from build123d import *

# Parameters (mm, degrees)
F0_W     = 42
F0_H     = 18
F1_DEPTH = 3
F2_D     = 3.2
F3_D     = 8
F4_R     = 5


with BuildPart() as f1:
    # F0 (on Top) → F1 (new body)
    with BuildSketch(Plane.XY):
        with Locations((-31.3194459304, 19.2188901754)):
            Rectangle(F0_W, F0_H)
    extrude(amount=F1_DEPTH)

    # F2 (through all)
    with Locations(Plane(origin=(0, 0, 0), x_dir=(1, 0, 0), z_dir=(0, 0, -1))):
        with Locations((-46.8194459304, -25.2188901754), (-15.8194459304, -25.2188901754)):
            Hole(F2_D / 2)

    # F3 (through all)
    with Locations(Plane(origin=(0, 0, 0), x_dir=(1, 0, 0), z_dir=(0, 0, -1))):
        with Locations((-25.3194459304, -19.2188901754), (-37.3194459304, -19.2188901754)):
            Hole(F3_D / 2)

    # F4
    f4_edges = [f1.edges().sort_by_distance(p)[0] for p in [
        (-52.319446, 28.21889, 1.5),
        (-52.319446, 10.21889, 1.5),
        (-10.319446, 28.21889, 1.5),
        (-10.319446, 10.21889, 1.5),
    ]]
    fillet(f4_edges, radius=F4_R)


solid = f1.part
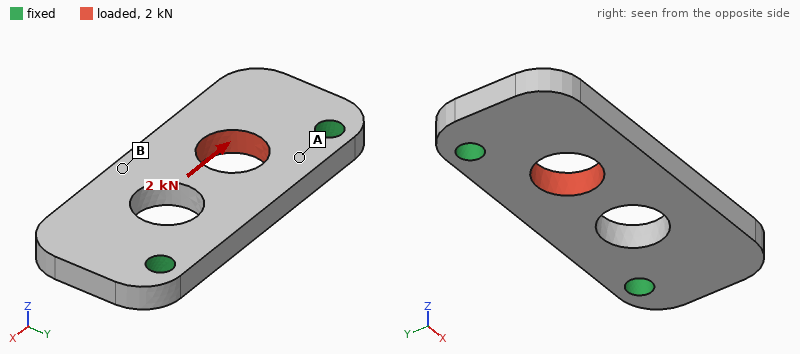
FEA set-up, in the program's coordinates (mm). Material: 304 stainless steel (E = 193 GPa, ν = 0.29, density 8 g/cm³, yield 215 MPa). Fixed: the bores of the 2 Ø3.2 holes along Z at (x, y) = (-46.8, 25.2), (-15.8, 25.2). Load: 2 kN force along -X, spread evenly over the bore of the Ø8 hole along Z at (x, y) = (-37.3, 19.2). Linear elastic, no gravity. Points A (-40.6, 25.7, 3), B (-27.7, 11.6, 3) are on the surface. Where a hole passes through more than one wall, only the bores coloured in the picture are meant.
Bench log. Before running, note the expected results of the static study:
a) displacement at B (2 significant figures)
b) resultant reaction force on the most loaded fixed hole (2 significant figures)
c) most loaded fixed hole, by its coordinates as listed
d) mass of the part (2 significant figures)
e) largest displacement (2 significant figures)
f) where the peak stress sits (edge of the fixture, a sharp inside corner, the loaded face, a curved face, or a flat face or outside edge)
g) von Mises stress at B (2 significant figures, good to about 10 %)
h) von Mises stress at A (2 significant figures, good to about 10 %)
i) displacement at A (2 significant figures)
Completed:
4.5 µm
1.3 kN
(-46.8, 25.2)
15 g
6.3 µm
edge of the fixture
20 MPa
48 MPa
1.4 µm
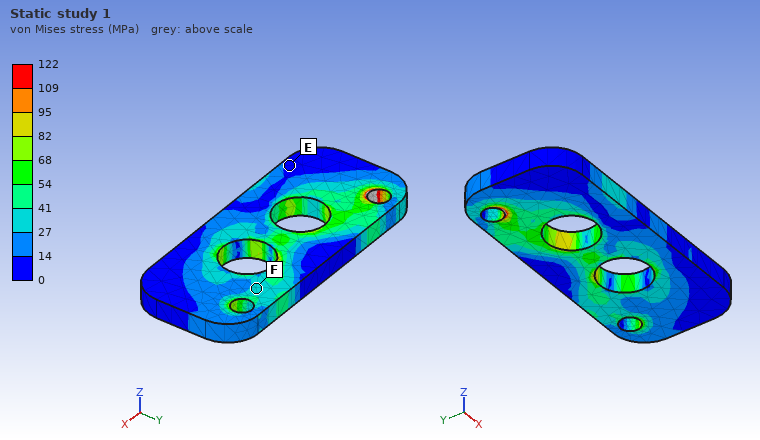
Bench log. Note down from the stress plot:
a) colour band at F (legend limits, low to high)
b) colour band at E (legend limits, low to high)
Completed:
27 to 41 MPa
0 to 14 MPa
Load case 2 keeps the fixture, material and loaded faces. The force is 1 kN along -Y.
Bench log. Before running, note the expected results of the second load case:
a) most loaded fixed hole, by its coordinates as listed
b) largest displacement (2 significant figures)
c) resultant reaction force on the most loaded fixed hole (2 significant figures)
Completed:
(-46.8, 25.2)
4.3 µm
740 N
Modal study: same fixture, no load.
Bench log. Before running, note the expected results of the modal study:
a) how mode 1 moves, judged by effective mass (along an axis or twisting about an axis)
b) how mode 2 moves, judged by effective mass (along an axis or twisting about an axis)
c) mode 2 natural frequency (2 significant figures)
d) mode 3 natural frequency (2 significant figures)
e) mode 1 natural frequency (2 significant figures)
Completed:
along Z
twisting about Y
13 kHz
16 kHz
7800 Hz
